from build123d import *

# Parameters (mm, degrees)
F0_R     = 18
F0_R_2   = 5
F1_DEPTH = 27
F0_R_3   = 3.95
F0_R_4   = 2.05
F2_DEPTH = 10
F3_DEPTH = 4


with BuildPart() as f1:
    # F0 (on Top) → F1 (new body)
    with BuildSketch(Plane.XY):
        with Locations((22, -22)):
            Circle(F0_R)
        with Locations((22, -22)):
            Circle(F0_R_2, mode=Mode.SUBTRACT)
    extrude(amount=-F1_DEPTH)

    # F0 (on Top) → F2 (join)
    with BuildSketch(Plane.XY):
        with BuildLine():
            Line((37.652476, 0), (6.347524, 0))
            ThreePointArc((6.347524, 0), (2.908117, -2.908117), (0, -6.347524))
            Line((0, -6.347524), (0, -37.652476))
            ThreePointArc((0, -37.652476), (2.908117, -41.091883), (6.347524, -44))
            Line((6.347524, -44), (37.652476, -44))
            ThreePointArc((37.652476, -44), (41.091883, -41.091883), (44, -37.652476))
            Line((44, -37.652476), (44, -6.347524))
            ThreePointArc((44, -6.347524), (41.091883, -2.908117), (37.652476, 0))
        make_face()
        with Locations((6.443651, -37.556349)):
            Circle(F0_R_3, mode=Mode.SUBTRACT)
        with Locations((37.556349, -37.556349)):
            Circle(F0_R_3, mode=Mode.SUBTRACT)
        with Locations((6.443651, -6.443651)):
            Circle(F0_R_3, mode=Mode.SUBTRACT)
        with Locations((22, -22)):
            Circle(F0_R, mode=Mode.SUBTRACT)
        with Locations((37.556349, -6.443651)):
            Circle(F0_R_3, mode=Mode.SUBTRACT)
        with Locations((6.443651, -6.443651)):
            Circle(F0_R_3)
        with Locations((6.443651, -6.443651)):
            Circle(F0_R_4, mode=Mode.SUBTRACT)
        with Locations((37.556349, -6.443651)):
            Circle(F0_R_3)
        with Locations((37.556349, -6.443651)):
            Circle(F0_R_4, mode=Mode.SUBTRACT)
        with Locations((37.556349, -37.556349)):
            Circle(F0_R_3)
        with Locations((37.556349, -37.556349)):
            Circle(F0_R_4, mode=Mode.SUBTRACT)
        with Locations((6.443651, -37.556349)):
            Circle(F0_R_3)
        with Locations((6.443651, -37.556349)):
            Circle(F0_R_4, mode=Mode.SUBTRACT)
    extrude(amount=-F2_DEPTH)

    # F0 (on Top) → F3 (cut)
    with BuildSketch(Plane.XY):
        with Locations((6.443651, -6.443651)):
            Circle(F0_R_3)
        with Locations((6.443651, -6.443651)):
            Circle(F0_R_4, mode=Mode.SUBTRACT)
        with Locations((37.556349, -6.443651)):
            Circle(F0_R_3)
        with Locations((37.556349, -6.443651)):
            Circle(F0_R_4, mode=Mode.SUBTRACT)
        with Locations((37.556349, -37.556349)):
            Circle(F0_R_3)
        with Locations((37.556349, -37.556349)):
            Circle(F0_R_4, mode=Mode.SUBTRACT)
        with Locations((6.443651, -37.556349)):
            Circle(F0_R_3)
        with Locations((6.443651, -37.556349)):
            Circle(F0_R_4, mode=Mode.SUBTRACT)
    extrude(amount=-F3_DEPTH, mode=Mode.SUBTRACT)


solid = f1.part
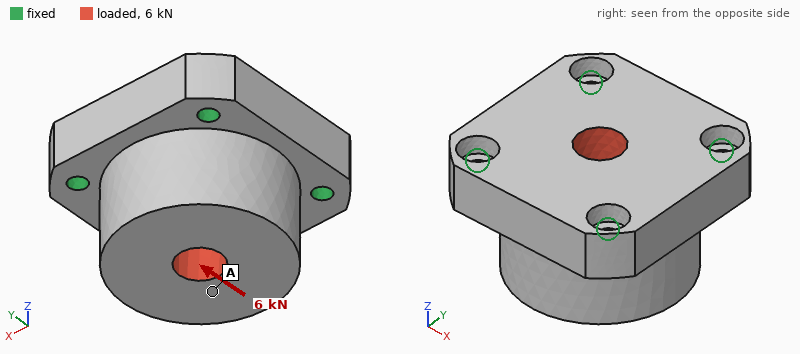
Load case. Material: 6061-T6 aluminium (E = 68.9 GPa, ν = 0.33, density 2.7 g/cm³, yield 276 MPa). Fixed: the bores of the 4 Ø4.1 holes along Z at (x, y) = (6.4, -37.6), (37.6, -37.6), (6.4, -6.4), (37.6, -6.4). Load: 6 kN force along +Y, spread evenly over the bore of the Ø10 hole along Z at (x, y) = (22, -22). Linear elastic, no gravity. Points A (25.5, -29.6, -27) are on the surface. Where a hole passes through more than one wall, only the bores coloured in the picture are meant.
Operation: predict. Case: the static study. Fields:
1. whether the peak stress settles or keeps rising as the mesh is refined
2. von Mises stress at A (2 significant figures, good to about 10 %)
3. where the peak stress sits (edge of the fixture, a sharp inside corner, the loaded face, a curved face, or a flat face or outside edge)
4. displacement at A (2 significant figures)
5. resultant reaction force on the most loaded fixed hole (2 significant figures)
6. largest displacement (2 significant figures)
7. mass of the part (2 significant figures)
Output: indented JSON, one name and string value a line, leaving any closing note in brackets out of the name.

{
  "whether the peak stress settles or keeps rising as the mesh is refined": "keeps rising",
  "von Mises stress at A": "7.1 MPa",
  "where the peak stress sits": "edge of the fixture",
  "displacement at A": "8.4 µm",
  "resultant reaction force on the most loaded fixed hole": "1.7 kN",
  "largest displacement": "8.9 µm",
  "mass of the part": "88 g"
}
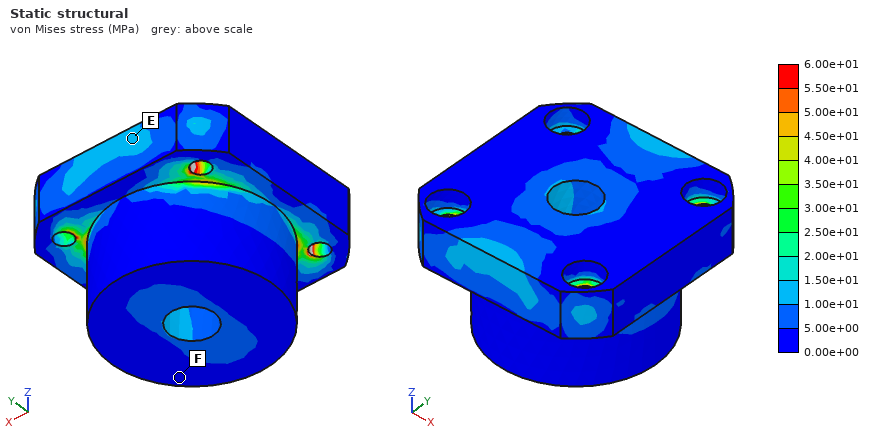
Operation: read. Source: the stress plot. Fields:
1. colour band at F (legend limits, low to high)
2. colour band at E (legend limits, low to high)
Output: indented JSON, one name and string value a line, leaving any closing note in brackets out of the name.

{
  "colour band at F": "0.00e+00 to 5.00e+00 MPa",
  "colour band at E": "1.00e+01 to 1.50e+01 MPa"
}
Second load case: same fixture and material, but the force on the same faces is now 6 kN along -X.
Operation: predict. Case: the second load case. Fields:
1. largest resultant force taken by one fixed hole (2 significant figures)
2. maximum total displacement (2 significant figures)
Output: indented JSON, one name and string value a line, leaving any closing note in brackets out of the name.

{
  "largest resultant force taken by one fixed hole": "1.7 kN",
  "maximum total displacement": "8.9 µm"
}
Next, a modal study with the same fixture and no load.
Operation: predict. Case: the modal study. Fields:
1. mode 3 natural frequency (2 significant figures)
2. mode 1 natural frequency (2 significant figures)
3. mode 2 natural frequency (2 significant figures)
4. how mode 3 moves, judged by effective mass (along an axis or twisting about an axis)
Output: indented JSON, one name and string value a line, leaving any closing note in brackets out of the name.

{
  "mode 3 natural frequency": "19 kHz",
  "mode 1 natural frequency": "18 kHz",
  "mode 2 natural frequency": "18 kHz",
  "how mode 3 moves, judged by effective mass": "along Z"
}
